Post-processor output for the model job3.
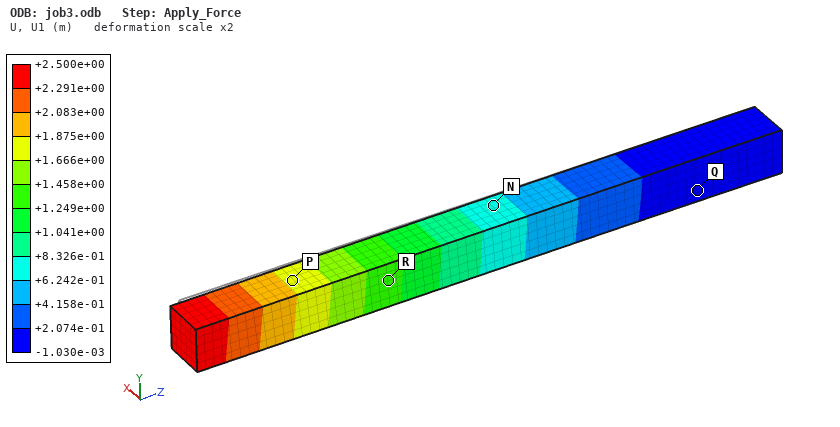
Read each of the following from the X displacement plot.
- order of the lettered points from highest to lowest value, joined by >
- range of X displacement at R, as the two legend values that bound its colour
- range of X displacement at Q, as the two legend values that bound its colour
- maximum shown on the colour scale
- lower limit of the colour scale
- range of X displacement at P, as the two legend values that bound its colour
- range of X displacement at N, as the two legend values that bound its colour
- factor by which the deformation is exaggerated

P > R > N > Q
+1.249e+00 to +1.458e+00 m
-1.030e-03 to +2.074e-01 m
+2.500e+00 m
-1.030e-03 m
+1.666e+00 to +1.875e+00 m
+6.242e-01 to +8.326e-01 m
2
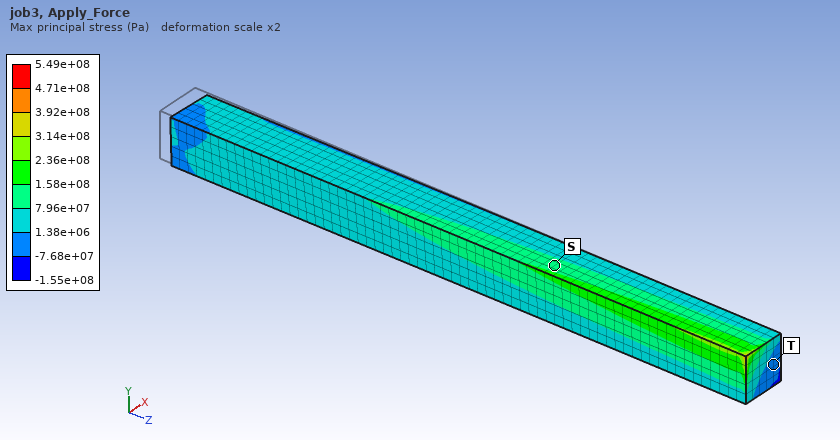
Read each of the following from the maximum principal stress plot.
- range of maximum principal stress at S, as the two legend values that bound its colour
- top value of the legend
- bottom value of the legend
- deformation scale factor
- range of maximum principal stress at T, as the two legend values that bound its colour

7.96e+07 to 1.58e+08 Pa
5.49e+08 Pa
-1.55e+08 Pa
2
-7.68e+07 to 1.38e+06 Pa
